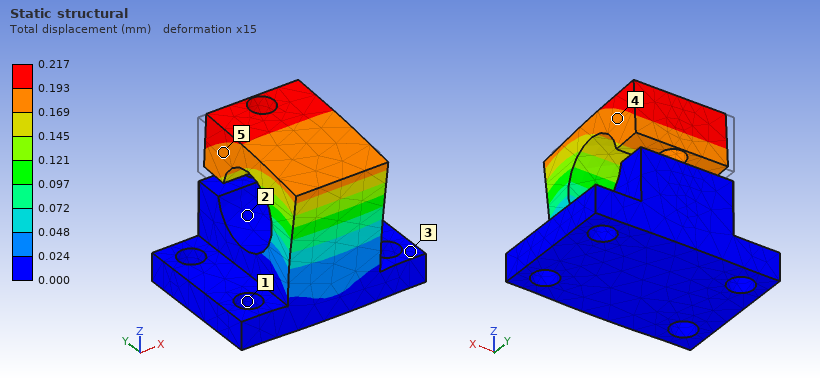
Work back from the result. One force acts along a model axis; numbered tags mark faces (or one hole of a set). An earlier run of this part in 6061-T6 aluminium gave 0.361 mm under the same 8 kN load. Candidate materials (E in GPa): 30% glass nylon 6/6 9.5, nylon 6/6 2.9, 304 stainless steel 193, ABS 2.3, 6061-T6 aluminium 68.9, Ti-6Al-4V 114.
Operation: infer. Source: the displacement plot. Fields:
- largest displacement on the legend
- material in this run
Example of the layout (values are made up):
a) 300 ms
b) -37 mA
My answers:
a) 0.217 mm
b) Ti-6Al-4V
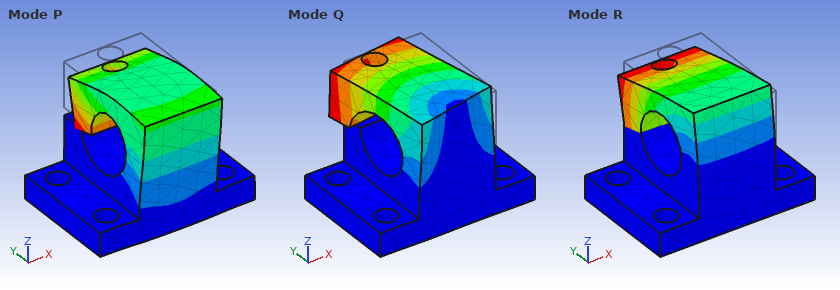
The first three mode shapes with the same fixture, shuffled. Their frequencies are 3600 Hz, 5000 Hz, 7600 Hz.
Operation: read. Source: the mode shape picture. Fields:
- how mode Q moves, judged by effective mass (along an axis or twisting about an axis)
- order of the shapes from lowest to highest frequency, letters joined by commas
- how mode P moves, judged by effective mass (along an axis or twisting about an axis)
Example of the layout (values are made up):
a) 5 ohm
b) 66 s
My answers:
a) along X
b) R, Q, P
c) along Y
